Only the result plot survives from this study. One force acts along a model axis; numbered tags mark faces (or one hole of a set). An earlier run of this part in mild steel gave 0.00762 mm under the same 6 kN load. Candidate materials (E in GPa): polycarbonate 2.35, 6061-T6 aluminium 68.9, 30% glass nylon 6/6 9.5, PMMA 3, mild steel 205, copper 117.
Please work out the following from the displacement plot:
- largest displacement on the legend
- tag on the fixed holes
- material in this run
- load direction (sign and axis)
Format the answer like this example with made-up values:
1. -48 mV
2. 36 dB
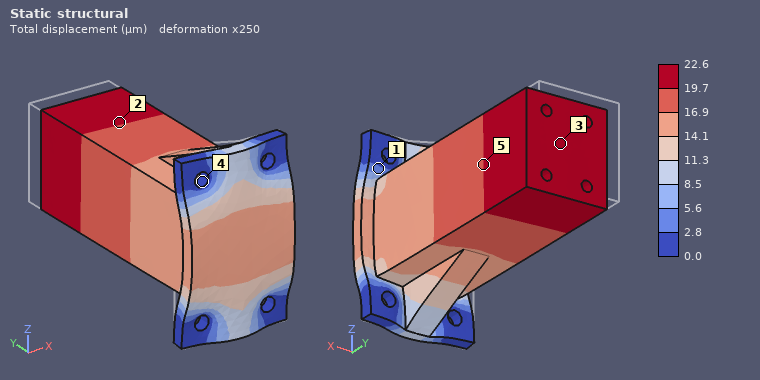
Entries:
1. 22.6 µm
2. 4
3. 6061-T6 aluminium
4. -Y
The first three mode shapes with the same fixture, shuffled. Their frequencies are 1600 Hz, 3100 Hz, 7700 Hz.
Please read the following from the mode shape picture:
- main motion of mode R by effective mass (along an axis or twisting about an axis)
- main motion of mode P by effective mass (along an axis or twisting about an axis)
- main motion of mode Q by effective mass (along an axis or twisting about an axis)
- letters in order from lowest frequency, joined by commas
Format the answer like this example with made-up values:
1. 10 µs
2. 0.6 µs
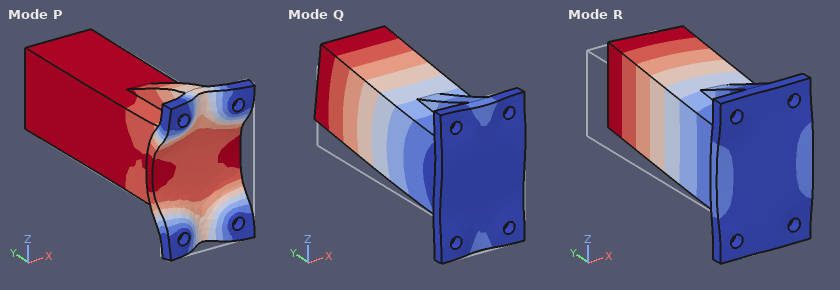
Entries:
1. along X
2. along Y
3. along Z
4. R, Q, P
